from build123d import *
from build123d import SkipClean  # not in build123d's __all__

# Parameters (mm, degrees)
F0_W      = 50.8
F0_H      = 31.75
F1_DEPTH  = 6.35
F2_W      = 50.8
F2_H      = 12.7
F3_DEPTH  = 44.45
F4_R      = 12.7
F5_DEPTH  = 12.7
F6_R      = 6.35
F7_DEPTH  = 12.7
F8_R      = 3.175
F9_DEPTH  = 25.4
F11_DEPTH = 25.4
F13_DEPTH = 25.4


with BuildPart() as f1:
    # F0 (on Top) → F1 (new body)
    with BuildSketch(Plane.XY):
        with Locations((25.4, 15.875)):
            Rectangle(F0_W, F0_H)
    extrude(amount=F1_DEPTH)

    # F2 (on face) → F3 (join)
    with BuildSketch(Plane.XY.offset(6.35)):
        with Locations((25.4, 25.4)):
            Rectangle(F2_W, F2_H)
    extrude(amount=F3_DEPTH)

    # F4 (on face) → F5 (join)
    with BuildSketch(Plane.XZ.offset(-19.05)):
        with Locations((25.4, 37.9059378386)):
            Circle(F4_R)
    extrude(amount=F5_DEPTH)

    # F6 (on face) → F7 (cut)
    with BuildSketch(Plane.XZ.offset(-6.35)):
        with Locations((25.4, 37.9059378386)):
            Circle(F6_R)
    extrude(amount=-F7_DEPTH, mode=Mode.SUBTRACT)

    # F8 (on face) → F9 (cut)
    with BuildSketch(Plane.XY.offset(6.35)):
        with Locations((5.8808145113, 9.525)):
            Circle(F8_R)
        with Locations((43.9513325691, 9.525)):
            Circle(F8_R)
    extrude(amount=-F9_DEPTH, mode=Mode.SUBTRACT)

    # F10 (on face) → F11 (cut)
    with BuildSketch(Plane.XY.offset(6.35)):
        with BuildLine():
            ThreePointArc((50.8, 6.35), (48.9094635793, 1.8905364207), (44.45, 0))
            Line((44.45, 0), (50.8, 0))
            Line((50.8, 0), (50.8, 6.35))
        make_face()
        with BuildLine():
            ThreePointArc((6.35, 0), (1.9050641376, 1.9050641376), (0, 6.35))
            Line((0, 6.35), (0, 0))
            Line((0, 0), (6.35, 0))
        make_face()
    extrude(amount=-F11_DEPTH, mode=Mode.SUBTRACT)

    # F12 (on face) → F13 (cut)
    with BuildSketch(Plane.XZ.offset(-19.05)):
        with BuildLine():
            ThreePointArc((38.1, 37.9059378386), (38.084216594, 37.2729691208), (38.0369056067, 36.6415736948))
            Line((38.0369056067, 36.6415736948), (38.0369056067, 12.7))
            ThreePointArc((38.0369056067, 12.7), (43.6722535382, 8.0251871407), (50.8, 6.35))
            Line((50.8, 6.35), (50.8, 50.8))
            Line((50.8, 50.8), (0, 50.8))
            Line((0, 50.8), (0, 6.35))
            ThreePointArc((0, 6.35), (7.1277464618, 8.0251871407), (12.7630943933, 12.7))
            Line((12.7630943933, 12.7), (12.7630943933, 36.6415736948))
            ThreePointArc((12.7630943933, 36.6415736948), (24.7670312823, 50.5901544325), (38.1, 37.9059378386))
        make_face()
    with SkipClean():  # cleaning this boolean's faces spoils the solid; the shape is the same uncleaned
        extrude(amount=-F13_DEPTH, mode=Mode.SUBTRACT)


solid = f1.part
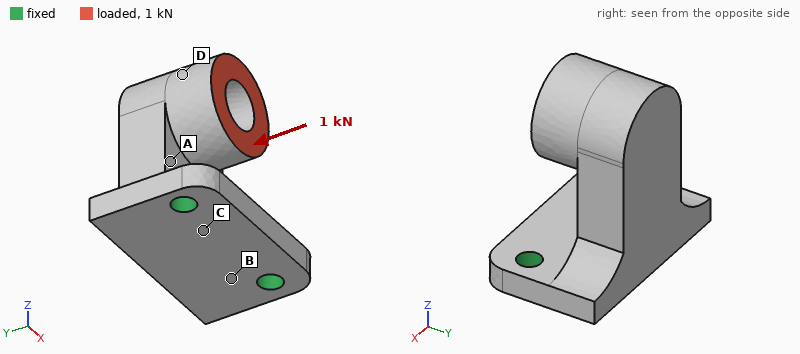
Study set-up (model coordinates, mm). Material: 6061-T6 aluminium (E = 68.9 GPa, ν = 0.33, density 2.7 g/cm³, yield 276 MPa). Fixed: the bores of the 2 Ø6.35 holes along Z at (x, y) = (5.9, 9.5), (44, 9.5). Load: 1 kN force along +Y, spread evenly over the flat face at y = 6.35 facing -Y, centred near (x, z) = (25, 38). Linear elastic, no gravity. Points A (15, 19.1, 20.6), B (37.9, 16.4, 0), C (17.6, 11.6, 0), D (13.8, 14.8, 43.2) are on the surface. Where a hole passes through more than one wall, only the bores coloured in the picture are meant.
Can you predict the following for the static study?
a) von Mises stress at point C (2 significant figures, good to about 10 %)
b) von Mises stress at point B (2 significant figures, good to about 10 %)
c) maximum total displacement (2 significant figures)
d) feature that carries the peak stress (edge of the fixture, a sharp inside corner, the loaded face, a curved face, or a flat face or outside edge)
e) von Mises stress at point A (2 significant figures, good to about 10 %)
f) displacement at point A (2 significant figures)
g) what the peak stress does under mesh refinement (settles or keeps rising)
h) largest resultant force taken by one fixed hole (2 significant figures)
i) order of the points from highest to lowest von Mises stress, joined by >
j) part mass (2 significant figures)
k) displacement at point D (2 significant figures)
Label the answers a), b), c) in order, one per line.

a) 49 MPa
b) 85 MPa
c) 0.36 mm
d) edge of the fixture
e) 24 MPa
f) 0.12 mm
g) keeps rising
h) 560 N
i) B > C > A > D
j) 77 g
k) 0.29 mm
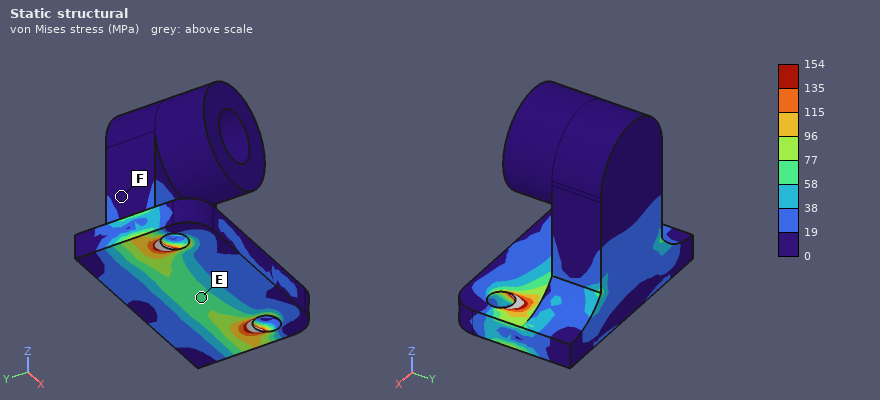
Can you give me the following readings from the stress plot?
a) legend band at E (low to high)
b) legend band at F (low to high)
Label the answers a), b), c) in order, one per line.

a) 58 to 77 MPa
b) 0 to 19 MPa
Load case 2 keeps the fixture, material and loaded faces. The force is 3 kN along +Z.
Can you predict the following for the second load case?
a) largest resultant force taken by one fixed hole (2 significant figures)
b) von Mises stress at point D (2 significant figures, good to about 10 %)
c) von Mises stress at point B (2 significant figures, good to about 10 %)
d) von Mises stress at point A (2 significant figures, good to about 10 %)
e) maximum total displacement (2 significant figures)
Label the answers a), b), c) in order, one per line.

a) 1.6 kN
b) 13 MPa
c) 79 MPa
d) 90 MPa
e) 0.44 mm
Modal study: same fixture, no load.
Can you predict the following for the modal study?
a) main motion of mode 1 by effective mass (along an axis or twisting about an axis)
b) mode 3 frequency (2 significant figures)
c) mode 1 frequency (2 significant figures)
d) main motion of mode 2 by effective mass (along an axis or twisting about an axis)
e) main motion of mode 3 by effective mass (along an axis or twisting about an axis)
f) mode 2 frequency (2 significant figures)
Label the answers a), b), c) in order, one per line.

a) along Y
b) 6500 Hz
c) 1600 Hz
d) along X
e) along Z
f) 3800 Hz
